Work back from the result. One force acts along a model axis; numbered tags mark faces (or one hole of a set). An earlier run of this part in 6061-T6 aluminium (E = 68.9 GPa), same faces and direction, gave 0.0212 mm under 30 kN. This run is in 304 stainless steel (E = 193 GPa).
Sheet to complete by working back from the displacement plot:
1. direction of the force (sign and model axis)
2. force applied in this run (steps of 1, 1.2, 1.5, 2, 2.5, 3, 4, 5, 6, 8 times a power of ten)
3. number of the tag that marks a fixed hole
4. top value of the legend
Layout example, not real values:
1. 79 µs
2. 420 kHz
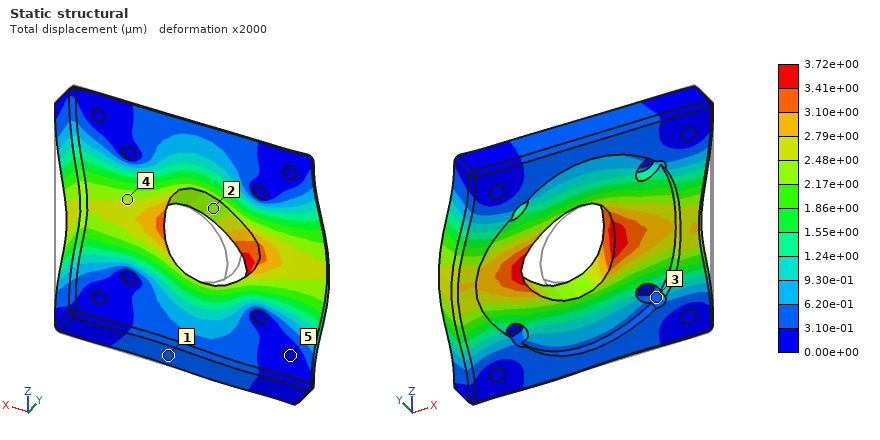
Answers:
1. -X
2. 15 kN
3. 5
4. 3.72e+00 µm
